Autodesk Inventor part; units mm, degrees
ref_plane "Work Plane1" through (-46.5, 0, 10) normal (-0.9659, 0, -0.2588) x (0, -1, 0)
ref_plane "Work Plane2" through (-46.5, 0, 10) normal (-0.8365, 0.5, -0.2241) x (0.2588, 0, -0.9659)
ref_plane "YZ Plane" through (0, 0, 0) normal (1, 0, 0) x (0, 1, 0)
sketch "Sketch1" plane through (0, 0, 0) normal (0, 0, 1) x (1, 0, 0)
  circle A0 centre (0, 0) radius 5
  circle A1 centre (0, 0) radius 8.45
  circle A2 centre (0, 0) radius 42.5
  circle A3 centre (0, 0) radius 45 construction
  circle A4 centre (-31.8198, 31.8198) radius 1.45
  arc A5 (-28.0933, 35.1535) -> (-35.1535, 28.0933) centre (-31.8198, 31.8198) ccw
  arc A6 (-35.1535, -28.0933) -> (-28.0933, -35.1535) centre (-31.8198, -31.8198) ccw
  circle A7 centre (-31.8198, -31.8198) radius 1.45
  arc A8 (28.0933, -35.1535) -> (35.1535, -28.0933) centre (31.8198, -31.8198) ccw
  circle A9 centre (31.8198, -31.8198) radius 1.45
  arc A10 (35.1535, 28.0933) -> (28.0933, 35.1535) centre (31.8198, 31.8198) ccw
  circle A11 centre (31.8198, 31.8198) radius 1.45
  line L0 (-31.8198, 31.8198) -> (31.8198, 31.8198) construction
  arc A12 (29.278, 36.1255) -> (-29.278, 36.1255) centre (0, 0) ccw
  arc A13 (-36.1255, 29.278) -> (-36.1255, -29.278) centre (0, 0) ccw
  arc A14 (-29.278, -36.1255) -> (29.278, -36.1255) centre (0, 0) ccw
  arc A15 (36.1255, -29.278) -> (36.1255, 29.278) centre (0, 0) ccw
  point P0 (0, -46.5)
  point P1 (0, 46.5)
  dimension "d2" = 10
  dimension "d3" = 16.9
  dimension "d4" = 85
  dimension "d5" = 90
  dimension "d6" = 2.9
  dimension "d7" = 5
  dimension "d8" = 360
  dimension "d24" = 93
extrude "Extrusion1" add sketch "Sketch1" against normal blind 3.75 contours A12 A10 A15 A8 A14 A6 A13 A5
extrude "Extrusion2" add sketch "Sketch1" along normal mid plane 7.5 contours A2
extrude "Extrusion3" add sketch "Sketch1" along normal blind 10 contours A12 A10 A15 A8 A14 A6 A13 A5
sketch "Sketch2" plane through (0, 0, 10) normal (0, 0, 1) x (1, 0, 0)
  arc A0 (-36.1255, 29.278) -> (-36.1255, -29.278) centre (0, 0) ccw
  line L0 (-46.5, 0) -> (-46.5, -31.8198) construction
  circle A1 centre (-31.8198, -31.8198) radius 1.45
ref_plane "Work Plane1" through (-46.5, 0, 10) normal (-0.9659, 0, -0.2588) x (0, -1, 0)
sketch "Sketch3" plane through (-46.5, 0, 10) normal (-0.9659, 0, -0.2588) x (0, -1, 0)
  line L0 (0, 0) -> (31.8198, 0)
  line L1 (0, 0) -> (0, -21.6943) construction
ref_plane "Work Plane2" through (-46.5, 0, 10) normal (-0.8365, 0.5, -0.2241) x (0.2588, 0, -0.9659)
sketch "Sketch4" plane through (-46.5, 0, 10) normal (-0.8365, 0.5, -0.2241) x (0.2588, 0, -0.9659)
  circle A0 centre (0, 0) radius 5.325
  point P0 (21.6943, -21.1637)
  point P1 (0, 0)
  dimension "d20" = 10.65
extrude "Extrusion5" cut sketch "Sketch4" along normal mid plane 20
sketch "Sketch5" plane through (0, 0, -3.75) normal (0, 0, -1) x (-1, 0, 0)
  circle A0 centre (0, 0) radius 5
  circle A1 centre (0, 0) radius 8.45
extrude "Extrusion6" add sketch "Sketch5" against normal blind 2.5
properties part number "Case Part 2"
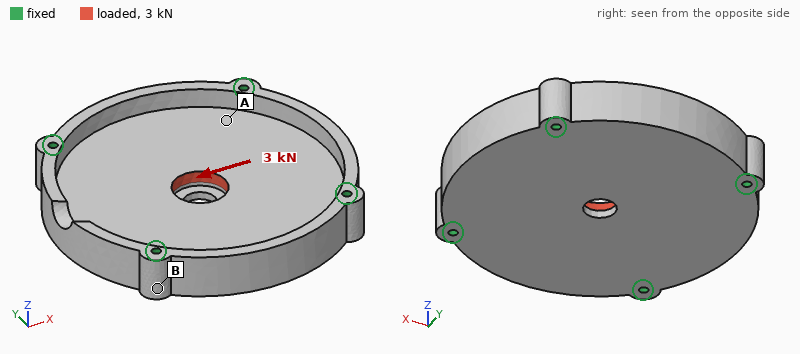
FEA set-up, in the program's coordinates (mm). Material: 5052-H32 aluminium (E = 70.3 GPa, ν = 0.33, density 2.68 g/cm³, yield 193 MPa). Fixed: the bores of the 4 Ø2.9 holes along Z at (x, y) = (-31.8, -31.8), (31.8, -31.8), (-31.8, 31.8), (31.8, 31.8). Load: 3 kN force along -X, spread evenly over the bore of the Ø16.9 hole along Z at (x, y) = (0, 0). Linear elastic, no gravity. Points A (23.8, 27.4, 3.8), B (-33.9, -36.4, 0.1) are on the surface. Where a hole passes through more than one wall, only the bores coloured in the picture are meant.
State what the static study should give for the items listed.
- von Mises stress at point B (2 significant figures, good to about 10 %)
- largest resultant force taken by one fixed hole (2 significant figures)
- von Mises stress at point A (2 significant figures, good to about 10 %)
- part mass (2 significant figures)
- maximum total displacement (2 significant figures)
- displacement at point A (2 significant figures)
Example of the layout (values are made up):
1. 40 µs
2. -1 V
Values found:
1. 3.0 MPa
2. 780 N
3. 7.3 MPa
4. 150 g
5. 5.4 µm
6. 1.1 µm
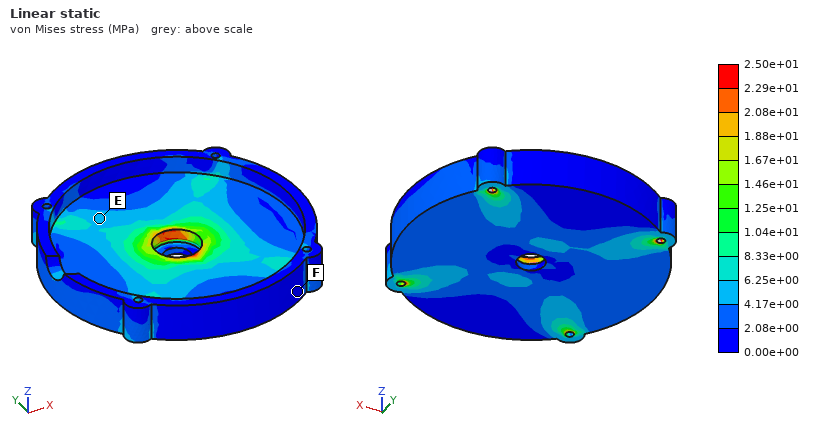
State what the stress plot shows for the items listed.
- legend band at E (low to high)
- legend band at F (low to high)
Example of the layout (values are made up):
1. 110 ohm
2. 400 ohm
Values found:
1. 4.17e+00 to 6.25e+00 MPa
2. 0.00e+00 to 2.08e+00 MPa
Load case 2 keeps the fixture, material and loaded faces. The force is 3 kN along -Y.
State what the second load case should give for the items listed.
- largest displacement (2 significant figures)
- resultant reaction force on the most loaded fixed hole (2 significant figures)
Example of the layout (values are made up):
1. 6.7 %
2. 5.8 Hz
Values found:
1. 5.4 µm
2. 770 N
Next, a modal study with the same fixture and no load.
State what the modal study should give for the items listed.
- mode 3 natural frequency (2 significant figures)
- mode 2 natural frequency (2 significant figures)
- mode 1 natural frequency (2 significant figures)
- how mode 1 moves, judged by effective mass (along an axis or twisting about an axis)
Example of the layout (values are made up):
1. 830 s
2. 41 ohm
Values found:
1. 10000 Hz
2. 9900 Hz
3. 6300 Hz
4. along Z
